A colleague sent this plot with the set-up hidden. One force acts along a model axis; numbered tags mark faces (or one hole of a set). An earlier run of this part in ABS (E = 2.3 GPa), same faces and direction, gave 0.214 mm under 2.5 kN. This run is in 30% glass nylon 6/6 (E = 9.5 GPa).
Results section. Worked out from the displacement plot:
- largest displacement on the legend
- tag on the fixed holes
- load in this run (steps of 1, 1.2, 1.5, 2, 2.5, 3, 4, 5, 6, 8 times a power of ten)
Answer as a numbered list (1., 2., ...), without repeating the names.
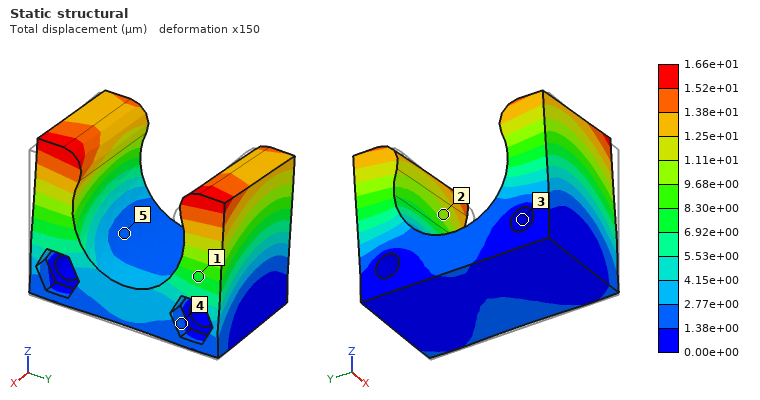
1. 1.66e+01 µm
2. 3
3. 800 N
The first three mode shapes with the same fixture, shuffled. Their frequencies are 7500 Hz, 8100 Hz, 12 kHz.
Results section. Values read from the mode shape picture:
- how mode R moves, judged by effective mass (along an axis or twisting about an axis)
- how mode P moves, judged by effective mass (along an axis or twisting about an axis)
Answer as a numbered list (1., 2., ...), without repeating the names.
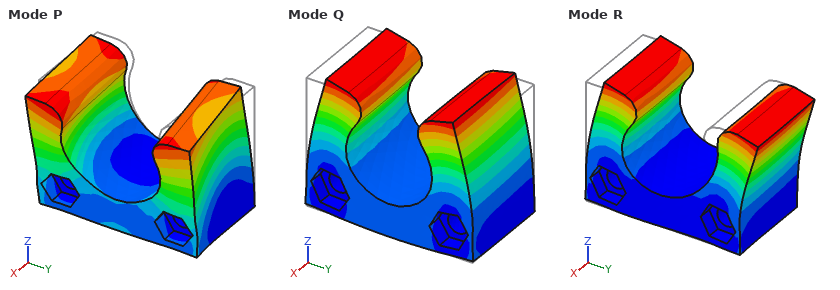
1. along Y
2. along X
